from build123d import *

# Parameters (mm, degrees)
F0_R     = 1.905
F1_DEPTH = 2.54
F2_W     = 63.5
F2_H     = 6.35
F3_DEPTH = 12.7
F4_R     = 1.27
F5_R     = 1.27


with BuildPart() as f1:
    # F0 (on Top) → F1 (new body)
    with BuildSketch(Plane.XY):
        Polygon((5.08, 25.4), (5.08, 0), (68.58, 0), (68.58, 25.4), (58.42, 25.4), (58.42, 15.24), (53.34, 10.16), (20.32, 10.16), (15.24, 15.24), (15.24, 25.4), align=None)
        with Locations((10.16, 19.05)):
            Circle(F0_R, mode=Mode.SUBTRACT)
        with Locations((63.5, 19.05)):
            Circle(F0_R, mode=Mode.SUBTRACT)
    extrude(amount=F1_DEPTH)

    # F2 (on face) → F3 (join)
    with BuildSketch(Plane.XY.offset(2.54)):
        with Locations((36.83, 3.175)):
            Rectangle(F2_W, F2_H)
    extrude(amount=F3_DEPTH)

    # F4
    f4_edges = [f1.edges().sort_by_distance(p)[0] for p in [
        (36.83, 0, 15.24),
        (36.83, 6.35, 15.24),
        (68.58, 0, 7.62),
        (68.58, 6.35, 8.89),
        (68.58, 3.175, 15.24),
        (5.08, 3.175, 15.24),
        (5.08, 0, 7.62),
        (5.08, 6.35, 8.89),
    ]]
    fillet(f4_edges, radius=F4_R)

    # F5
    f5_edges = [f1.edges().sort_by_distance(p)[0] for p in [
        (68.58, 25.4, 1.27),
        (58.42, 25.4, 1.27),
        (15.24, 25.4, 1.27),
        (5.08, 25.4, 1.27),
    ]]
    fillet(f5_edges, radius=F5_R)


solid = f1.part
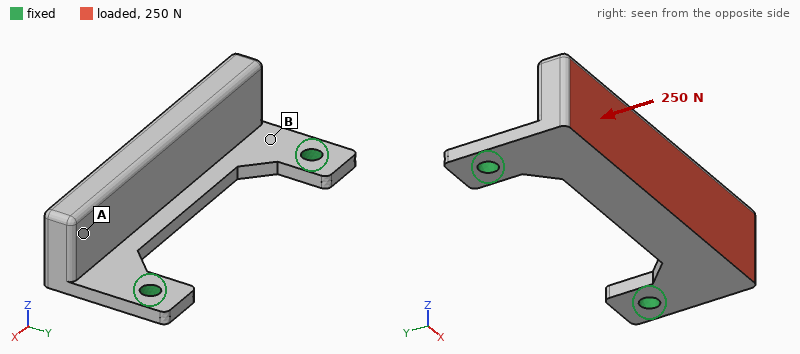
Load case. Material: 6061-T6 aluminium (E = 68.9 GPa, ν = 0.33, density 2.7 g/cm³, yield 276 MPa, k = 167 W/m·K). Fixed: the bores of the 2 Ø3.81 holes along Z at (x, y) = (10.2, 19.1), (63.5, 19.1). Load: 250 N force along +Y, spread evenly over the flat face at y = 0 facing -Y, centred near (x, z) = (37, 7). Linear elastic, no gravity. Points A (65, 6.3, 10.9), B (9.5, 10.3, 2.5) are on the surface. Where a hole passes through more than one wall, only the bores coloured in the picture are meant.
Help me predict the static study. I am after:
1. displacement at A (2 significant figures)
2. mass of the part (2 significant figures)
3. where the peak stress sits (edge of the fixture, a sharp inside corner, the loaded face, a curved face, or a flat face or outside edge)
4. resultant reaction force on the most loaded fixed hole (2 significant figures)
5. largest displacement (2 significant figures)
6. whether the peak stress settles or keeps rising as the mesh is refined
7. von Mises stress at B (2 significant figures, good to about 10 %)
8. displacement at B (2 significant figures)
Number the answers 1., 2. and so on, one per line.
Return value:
1. 0.085 mm
2. 20 g
3. edge of the fixture
4. 140 N
5. 0.14 mm
6. keeps rising
7. 49 MPa
8. 0.022 mm
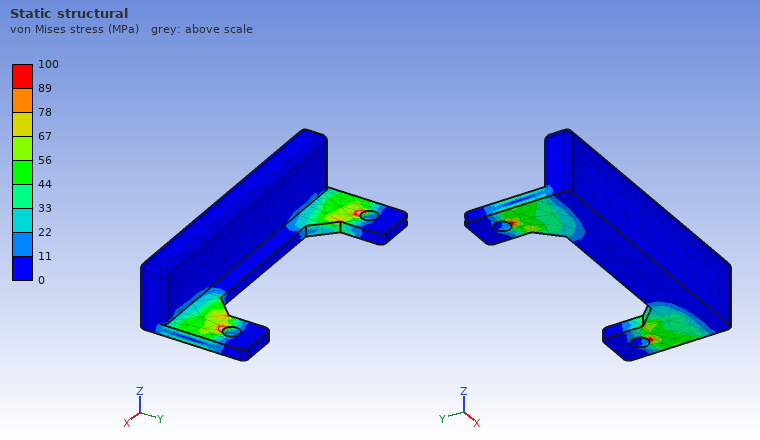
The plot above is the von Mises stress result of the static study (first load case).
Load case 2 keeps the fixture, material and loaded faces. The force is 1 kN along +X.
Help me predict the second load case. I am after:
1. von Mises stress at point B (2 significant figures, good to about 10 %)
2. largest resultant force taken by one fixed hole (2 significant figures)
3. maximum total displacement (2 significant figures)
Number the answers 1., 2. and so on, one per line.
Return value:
1. 28 MPa
2. 580 N
3. 39 µm
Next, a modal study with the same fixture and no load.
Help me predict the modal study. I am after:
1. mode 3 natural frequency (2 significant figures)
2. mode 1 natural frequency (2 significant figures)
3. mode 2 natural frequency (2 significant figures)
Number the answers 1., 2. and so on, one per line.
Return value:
1. 5900 Hz
2. 1400 Hz
3. 4500 Hz
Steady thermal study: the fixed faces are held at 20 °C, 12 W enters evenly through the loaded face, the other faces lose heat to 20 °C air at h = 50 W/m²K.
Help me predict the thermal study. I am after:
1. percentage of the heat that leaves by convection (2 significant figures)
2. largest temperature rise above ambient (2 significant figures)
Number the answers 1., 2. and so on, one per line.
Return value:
1. 16 %
2. 16 K
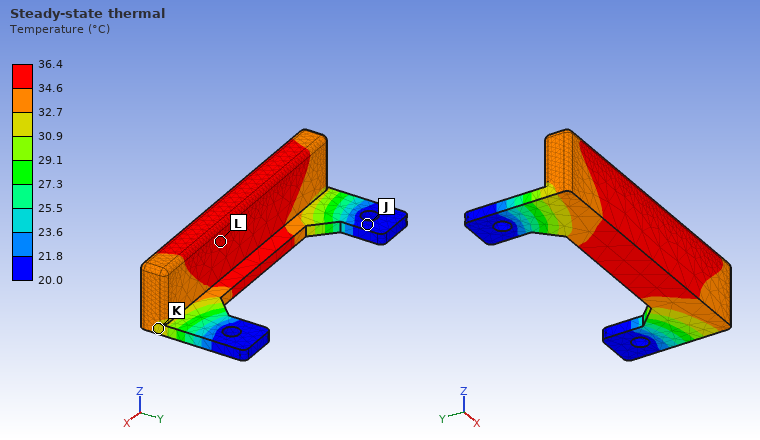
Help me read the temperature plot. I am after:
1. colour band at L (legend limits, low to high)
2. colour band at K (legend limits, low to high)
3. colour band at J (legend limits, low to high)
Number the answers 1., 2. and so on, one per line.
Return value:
1. 34.6 to 36.4 °C
2. 30.9 to 32.7 °C
3. 20.0 to 21.8 °C
